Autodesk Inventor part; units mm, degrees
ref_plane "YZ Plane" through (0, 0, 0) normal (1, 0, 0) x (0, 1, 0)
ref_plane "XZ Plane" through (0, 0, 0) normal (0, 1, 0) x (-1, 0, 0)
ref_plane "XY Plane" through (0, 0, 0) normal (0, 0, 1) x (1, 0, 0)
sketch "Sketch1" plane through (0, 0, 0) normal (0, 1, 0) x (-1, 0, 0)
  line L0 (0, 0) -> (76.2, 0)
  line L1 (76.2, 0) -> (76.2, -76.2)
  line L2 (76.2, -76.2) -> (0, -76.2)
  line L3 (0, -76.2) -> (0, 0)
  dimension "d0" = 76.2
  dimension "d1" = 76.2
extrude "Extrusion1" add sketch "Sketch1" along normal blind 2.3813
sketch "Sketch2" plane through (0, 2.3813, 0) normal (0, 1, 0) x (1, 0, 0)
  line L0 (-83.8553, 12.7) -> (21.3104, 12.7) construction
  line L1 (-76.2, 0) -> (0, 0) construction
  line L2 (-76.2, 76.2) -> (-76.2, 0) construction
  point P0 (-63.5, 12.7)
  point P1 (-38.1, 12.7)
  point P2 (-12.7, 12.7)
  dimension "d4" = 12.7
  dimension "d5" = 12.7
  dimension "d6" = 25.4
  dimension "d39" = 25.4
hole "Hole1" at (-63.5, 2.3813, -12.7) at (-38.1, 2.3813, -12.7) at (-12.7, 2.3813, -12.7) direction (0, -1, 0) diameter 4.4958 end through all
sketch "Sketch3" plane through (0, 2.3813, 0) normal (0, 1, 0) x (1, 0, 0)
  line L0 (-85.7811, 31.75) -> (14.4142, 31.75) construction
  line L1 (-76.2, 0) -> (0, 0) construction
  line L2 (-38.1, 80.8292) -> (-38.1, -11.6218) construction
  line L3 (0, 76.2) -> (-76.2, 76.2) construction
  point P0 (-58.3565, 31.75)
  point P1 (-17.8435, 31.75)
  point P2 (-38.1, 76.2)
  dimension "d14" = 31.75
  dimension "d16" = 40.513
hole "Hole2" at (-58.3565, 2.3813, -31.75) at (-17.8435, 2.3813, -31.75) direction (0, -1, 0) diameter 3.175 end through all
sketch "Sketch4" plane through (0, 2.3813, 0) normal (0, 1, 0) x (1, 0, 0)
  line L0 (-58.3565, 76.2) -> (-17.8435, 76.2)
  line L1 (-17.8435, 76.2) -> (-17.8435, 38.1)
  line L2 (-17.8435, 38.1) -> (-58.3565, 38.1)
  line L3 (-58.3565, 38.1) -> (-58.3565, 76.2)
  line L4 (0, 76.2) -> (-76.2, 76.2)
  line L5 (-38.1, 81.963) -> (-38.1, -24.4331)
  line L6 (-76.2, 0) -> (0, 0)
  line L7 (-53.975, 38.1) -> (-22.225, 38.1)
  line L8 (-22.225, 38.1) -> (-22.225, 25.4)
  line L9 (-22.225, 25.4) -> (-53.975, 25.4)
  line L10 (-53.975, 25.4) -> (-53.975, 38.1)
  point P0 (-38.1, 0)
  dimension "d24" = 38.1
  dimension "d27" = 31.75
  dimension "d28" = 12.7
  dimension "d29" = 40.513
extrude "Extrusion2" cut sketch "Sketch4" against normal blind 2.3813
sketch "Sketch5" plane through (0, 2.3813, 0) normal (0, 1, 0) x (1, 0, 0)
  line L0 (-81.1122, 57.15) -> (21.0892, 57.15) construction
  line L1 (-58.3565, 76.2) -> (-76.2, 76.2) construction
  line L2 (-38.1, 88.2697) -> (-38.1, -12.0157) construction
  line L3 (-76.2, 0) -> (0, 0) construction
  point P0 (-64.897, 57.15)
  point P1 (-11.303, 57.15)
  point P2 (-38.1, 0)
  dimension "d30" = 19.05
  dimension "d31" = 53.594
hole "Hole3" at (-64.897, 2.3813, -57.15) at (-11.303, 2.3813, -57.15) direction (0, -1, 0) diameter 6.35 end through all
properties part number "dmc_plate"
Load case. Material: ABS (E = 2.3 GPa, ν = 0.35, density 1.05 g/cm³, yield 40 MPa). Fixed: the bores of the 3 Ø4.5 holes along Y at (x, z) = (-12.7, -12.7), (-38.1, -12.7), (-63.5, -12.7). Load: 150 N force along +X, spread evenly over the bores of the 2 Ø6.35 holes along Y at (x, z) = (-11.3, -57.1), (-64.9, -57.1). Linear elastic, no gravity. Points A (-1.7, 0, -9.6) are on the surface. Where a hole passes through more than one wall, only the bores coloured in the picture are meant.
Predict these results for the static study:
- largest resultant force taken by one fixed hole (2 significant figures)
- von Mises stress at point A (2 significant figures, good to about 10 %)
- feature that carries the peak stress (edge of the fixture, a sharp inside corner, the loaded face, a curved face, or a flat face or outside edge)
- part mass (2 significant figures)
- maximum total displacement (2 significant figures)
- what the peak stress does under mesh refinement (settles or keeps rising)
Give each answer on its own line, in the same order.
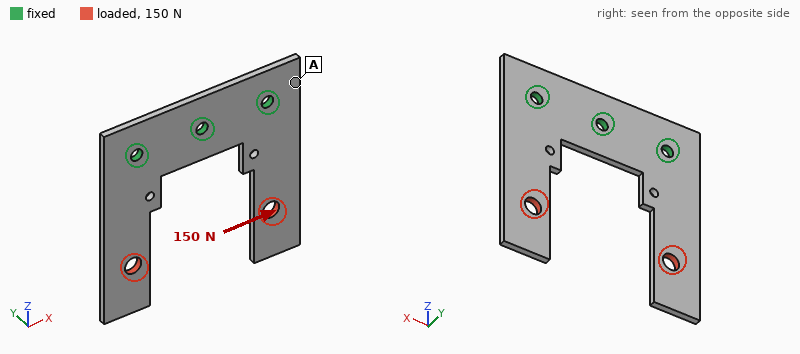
110 N
3.3 MPa
a sharp inside corner
9.3 g
1.0 mm
keeps rising
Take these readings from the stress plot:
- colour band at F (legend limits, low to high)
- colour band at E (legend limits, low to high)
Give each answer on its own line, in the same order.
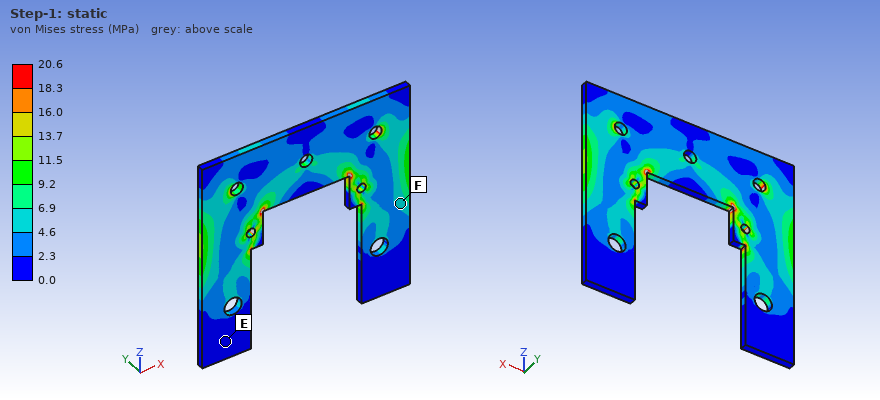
4.6 to 6.9 MPa
0.0 to 2.3 MPa
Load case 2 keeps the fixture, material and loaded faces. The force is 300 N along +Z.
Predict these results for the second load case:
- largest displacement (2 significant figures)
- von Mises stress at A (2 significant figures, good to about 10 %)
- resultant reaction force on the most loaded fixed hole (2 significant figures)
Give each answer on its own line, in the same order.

0.12 mm
1.1 MPa
150 N
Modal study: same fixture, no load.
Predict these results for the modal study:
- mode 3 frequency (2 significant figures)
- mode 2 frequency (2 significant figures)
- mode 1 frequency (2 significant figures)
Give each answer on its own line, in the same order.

880 Hz
170 Hz
170 Hz
